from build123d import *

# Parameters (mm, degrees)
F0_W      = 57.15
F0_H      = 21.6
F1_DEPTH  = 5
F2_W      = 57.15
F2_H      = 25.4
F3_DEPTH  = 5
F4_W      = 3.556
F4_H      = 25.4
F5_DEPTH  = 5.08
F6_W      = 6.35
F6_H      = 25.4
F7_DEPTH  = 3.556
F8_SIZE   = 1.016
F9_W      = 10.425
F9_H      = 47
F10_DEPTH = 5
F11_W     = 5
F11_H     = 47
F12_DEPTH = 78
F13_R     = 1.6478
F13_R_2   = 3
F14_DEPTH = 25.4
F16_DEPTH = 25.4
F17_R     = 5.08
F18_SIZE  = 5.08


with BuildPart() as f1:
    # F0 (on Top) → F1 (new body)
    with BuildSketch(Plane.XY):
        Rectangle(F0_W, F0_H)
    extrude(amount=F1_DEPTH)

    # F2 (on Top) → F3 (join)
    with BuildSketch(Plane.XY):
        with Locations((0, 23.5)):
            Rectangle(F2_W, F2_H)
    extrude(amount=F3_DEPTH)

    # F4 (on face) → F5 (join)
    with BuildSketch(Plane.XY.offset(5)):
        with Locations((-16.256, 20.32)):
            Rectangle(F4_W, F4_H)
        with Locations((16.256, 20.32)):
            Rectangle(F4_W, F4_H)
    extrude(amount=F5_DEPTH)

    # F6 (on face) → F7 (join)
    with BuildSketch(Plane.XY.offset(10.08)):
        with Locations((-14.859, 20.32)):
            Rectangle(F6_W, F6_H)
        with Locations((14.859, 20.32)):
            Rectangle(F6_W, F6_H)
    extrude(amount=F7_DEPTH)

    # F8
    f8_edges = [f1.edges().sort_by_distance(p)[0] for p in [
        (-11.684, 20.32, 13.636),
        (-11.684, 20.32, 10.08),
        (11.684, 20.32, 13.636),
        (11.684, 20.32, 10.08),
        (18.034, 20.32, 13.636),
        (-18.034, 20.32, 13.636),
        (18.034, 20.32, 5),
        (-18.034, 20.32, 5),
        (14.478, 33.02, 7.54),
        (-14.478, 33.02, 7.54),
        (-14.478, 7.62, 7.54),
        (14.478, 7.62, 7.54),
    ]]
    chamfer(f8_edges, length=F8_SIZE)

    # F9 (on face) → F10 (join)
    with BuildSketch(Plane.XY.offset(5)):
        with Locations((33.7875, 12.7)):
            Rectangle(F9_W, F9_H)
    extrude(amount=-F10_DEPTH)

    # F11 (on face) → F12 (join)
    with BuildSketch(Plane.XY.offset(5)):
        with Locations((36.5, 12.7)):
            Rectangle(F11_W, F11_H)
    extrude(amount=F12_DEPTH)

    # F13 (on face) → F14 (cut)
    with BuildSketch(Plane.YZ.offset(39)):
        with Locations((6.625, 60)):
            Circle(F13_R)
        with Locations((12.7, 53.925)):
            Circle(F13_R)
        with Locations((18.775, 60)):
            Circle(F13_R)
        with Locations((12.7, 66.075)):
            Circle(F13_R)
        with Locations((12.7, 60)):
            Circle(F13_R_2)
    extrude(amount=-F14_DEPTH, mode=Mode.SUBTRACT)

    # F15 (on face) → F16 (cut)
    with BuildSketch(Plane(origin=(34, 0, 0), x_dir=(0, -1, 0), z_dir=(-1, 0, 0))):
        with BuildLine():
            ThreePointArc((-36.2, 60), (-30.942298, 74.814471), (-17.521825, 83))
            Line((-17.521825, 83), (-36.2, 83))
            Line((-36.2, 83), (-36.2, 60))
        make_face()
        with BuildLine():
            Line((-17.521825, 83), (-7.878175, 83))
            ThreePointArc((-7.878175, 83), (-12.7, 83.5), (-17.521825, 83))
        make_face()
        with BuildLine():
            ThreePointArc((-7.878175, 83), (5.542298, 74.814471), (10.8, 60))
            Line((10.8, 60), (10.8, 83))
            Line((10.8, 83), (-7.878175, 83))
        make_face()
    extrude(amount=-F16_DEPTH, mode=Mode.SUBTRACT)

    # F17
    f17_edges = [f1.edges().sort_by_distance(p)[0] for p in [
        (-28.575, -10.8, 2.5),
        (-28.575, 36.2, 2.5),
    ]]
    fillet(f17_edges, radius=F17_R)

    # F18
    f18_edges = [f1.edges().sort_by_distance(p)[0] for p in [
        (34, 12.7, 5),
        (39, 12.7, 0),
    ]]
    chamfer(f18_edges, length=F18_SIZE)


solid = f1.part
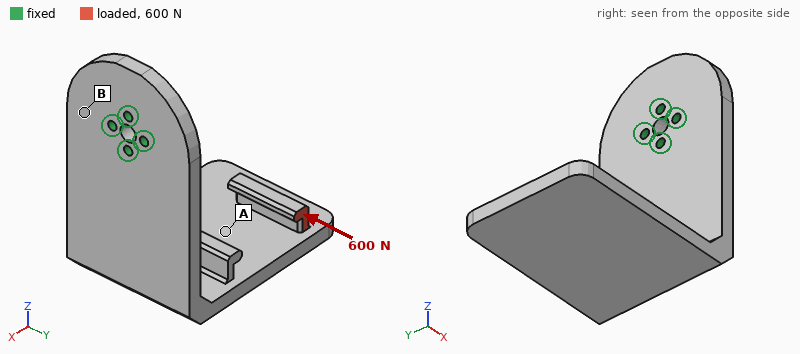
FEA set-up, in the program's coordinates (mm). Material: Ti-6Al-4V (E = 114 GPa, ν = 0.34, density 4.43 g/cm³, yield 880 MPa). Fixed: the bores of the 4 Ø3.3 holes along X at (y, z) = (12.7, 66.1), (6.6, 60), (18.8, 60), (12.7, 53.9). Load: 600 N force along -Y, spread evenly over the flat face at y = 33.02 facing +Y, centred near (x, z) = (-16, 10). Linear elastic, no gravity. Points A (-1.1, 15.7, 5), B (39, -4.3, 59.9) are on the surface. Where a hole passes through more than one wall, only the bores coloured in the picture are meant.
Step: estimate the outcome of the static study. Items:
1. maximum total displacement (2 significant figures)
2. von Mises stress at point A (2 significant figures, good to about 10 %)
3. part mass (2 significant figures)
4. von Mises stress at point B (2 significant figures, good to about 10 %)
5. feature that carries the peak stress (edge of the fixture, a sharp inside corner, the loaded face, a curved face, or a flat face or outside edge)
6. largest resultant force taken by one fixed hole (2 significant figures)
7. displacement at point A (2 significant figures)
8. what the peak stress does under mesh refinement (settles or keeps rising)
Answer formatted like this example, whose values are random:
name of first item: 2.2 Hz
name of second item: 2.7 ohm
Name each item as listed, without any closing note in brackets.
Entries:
maximum total displacement: 1.2 mm
von Mises stress at point A: 29 MPa
part mass: 150 g
von Mises stress at point B: 94 MPa
feature that carries the peak stress: edge of the fixture
largest resultant force taken by one fixed hole: 1.4 kN
displacement at point A: 0.67 mm
what the peak stress does under mesh refinement: keeps rising
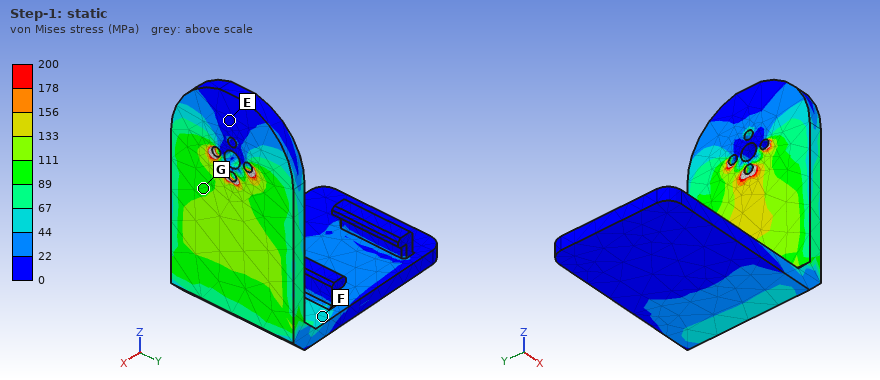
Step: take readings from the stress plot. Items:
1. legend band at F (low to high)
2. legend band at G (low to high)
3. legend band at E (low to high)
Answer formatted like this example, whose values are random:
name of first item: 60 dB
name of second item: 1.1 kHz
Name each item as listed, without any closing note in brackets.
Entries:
legend band at F: 44 to 67 MPa
legend band at G: 89 to 111 MPa
legend band at E: 0 to 22 MPa
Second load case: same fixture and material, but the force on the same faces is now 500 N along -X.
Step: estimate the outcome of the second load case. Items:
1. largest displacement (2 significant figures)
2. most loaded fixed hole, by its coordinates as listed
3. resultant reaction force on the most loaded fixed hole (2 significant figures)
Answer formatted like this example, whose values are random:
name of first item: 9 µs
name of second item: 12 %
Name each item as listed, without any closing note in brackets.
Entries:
largest displacement: 0.77 mm
most loaded fixed hole, by its coordinates as listed: (12.7, 53.9)
resultant reaction force on the most loaded fixed hole: 1.4 kN
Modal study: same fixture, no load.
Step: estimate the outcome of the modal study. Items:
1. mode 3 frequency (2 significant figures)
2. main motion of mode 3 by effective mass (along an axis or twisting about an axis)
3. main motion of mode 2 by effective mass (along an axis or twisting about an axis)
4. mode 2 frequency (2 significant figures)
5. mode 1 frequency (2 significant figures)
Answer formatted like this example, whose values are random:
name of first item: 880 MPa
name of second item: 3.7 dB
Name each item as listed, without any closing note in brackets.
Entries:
mode 3 frequency: 1100 Hz
main motion of mode 3 by effective mass: along X
main motion of mode 2 by effective mass: along Y
mode 2 frequency: 600 Hz
mode 1 frequency: 380 Hz
